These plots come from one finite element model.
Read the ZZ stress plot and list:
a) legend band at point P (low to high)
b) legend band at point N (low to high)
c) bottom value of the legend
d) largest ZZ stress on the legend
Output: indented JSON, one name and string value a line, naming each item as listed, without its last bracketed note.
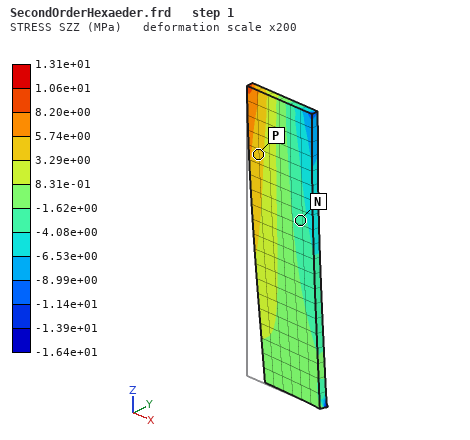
{
  "legend band at point P": "3.29e+00 to 5.74e+00 MPa",
  "legend band at point N": "-4.08e+00 to -1.62e+00 MPa",
  "bottom value of the legend": "-1.64e+01 MPa",
  "largest ZZ stress on the legend": "1.31e+01 MPa"
}
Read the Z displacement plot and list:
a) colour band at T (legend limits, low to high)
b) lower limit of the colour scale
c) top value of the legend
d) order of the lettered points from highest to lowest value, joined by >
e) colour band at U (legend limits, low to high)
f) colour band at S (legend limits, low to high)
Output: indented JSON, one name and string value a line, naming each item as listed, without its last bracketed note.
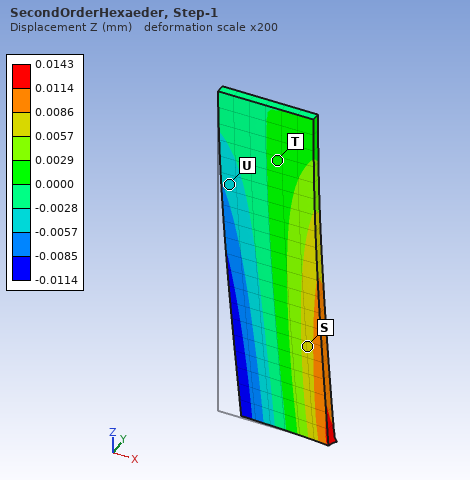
{
  "colour band at T": "0.0000 to 0.0029 mm",
  "lower limit of the colour scale": "-0.0114 mm",
  "top value of the legend": "0.0143 mm",
  "order of the lettered points from highest to lowest value, joined by >": "S > T > U",
  "colour band at U": "-0.0057 to -0.0028 mm",
  "colour band at S": "0.0057 to 0.0086 mm"
}
